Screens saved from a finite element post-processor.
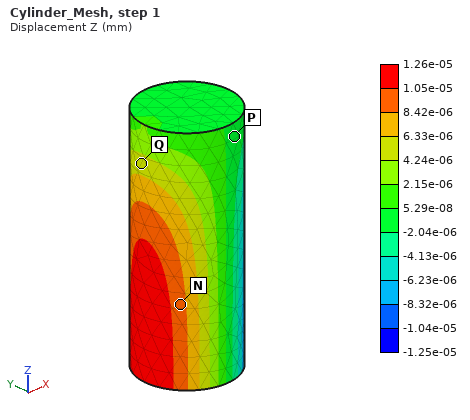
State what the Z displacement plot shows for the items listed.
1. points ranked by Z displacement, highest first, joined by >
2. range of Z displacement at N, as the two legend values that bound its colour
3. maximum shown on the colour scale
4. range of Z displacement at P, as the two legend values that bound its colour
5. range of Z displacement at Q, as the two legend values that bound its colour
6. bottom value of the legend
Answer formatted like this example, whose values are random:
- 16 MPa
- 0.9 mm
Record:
- N > Q > P
- 8.42e-06 to 1.05e-05 mm
- 1.26e-05 mm
- -2.04e-06 to 5.29e-08 mm
- 4.24e-06 to 6.33e-06 mm
- -1.25e-05 mm
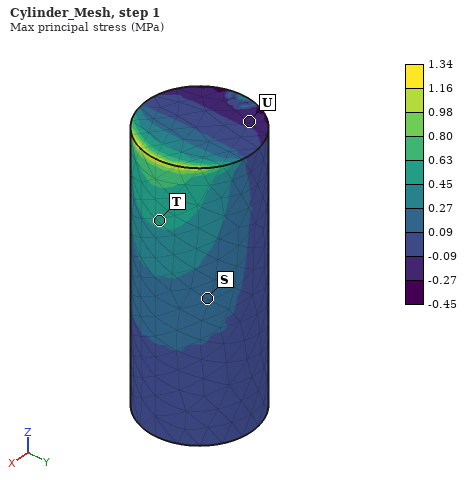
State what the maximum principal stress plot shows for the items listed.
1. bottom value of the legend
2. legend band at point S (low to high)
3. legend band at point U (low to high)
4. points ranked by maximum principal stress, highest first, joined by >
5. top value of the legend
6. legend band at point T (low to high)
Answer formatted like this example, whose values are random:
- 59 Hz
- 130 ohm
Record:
- -0.45 MPa
- 0.09 to 0.27 MPa
- -0.27 to -0.09 MPa
- T > S > U
- 1.34 MPa
- 0.45 to 0.63 MPa
